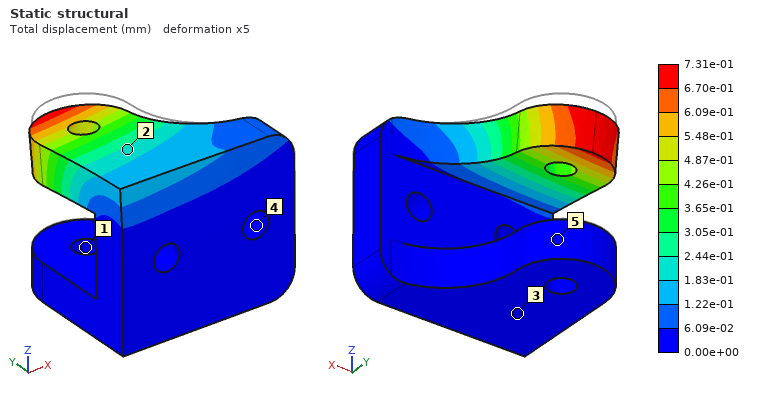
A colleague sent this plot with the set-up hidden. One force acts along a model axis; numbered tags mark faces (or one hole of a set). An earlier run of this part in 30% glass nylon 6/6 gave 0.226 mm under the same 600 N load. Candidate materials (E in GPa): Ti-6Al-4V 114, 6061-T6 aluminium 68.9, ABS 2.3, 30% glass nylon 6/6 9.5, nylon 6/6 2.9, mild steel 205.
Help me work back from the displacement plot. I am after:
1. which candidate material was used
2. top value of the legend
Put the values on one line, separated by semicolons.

nylon 6/6; 7.31e-01 mm
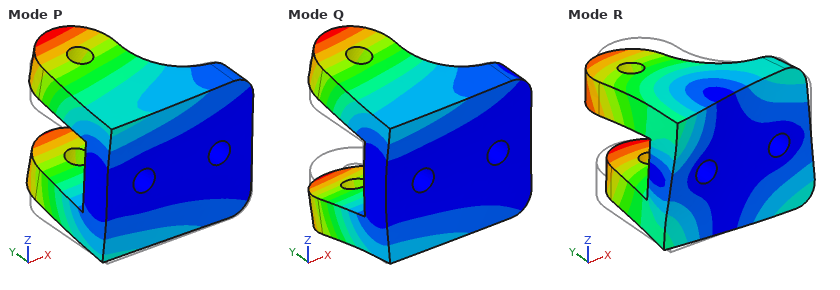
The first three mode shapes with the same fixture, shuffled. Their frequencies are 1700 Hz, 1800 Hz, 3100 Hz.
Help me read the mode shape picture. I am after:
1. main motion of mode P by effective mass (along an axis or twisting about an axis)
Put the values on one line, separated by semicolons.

along Z
